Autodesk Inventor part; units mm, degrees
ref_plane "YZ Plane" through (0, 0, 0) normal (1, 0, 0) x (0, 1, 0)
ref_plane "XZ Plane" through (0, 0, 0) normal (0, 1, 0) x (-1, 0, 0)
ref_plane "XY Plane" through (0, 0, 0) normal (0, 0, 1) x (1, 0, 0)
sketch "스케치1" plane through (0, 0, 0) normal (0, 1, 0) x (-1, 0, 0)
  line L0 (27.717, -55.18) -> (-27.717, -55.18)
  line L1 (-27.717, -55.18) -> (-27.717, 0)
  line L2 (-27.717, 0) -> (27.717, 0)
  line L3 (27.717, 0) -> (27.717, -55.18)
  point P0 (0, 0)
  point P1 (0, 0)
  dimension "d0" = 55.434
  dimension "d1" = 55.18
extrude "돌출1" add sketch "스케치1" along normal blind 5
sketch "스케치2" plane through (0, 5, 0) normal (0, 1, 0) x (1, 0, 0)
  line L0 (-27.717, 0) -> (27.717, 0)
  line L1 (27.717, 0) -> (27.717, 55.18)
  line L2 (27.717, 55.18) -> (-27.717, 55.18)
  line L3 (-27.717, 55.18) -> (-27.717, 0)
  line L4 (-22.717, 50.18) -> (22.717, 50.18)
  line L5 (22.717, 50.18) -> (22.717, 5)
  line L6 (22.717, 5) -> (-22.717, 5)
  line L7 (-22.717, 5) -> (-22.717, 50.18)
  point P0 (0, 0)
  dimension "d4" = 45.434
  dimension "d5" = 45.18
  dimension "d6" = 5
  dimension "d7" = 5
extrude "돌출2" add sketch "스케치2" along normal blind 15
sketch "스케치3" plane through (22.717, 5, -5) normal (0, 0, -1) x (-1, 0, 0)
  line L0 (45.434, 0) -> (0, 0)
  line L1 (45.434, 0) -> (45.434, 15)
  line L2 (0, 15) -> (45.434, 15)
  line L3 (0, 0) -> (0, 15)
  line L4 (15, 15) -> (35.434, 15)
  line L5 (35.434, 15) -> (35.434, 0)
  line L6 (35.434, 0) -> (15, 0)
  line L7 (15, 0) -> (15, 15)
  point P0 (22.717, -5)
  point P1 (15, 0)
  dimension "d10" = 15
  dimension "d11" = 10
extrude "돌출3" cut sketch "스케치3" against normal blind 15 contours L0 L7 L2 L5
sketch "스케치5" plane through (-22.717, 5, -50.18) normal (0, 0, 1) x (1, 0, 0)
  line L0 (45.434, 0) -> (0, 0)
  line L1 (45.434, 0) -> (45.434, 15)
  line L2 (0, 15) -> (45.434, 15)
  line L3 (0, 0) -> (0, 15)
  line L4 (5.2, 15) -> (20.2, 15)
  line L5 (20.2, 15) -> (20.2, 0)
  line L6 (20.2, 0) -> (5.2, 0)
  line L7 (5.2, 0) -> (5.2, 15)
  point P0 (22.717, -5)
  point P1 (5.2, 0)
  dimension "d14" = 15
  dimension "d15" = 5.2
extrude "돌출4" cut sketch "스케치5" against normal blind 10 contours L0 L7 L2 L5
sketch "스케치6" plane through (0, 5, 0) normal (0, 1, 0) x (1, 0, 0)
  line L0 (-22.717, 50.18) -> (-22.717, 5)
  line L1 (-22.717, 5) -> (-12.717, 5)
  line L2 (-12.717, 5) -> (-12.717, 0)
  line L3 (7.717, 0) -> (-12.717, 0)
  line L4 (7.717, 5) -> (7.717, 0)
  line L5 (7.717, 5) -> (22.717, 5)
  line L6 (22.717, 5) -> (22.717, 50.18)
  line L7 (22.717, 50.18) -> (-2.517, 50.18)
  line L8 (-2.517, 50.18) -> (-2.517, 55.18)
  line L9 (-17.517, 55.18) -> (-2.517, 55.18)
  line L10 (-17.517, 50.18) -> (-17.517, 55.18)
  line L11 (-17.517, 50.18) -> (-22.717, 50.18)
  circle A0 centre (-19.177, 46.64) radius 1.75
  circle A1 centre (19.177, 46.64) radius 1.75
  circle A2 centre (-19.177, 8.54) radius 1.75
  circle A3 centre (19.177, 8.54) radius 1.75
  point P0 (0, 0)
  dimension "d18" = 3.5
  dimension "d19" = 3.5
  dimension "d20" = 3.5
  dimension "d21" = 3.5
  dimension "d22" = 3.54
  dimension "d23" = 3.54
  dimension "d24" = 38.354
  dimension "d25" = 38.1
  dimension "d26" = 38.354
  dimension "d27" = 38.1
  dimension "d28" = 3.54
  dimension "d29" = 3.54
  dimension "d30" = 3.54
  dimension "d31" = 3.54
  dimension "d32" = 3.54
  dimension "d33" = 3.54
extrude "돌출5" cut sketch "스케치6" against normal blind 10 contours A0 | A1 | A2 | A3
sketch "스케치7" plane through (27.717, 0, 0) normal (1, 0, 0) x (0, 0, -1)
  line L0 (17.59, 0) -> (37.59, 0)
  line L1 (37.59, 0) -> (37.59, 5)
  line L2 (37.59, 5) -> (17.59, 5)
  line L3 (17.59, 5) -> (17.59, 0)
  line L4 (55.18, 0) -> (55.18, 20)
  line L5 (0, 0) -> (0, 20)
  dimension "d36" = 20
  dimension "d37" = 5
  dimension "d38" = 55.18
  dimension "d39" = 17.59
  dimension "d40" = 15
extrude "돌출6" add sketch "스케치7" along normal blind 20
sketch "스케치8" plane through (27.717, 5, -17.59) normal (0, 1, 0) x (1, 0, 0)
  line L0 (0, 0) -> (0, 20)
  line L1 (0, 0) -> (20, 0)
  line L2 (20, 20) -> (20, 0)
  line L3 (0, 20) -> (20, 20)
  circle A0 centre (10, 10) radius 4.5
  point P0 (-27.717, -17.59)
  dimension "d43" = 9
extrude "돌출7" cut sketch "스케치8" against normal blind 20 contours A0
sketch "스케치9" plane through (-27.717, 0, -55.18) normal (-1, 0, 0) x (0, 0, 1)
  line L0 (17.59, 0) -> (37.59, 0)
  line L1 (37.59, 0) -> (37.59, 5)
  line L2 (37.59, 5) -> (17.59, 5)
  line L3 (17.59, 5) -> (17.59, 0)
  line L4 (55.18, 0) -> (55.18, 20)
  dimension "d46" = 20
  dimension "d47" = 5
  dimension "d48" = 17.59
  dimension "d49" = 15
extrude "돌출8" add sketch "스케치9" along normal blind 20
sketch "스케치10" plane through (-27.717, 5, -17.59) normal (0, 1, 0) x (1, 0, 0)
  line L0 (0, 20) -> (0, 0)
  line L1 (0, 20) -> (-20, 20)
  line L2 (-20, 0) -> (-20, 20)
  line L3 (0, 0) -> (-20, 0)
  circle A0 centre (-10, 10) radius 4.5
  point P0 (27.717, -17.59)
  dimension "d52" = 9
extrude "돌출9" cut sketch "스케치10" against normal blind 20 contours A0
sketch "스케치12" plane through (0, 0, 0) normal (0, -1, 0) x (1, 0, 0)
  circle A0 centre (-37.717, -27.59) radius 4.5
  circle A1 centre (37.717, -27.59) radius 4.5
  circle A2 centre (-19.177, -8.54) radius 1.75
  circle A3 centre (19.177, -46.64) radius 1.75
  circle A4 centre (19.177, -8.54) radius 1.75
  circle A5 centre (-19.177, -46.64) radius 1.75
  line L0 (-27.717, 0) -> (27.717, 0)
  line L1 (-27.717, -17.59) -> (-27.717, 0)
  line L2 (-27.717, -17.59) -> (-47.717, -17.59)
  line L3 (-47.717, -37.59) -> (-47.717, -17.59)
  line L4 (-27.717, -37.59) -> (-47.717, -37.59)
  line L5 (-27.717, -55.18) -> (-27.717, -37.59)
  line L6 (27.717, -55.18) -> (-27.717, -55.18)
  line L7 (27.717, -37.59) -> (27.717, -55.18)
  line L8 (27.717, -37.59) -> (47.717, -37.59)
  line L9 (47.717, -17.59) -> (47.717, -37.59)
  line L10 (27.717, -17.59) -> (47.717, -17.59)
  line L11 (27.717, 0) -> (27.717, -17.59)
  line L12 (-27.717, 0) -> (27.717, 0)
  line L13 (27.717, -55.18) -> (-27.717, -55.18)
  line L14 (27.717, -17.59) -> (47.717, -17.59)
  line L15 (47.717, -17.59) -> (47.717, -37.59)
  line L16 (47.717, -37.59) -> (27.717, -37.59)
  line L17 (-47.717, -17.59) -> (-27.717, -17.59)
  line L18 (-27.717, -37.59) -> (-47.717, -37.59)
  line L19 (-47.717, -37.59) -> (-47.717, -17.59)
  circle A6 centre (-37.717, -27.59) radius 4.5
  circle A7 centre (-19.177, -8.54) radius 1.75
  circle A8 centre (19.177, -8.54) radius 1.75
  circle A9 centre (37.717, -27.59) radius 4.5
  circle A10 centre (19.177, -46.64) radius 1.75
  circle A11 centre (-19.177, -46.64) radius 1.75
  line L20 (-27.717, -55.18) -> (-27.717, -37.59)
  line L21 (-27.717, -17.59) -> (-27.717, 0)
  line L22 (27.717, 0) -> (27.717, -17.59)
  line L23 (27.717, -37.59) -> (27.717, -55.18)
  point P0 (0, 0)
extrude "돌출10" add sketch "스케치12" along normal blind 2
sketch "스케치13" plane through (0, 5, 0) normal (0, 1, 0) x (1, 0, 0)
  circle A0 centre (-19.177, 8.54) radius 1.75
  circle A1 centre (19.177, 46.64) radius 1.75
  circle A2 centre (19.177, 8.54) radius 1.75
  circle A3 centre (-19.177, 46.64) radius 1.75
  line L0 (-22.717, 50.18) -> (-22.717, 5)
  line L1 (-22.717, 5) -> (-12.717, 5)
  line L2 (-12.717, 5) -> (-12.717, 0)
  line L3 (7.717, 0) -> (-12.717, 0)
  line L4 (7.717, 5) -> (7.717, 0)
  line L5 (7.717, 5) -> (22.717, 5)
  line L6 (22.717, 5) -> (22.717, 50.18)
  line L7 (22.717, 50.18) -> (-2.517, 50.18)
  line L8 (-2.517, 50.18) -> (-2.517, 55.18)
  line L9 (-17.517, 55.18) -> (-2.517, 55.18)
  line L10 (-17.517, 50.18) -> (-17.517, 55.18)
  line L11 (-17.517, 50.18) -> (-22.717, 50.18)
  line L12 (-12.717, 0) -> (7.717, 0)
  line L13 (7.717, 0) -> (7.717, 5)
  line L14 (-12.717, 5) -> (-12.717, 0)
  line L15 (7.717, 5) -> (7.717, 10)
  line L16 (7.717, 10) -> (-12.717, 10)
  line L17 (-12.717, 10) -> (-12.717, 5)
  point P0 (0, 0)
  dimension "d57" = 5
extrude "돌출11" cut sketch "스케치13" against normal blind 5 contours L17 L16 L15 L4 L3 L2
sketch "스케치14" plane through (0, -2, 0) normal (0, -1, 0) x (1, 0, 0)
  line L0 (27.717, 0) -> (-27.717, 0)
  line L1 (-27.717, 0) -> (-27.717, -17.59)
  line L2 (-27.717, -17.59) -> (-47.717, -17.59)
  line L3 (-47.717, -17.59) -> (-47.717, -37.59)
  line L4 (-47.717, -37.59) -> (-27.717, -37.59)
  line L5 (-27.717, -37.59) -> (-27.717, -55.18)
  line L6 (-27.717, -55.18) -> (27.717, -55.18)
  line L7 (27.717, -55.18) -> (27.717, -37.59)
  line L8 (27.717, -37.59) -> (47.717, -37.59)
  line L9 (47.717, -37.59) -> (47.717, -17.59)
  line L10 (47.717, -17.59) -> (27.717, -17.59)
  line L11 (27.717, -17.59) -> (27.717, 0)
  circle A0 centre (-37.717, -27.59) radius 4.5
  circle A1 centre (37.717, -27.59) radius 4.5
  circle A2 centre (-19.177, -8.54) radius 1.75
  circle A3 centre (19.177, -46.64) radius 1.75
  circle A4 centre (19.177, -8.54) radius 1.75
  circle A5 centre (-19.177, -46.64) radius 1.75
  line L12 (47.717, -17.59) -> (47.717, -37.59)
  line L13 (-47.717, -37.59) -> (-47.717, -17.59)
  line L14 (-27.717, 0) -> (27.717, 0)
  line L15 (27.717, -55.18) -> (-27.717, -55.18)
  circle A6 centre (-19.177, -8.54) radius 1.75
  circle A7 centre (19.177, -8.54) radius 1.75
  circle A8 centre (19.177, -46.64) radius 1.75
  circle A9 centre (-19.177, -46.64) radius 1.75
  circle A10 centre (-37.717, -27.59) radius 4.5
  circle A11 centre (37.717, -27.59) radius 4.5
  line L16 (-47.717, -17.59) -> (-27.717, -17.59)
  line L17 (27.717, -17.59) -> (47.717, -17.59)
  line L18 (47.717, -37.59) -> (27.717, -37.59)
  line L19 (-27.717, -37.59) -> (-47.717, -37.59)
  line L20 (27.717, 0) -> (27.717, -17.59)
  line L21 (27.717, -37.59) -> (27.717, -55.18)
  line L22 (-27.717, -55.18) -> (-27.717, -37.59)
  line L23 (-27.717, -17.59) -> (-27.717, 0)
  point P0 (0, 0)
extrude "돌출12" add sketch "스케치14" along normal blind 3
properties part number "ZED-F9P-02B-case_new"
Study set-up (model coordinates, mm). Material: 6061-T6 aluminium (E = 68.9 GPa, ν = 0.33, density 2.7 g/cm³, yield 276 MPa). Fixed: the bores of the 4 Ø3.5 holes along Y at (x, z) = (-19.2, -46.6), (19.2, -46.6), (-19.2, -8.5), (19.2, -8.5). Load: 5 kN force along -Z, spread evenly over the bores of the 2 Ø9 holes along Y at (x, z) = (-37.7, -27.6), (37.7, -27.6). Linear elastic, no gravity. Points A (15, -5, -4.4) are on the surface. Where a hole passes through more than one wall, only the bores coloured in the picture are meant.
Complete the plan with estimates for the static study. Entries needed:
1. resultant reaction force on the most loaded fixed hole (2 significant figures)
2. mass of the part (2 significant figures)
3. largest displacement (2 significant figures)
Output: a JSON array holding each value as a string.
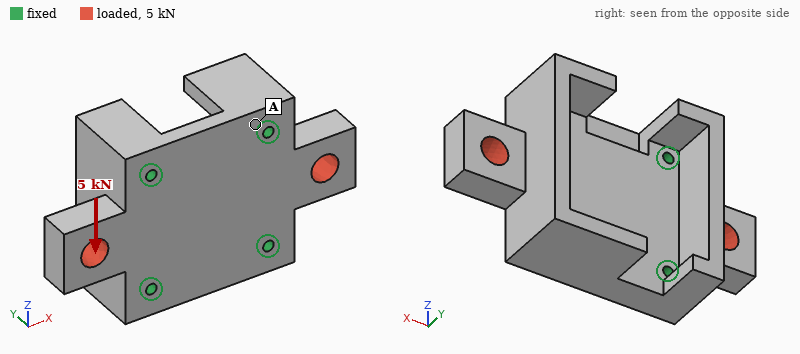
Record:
["1.6 kN", "130 g", "30 µm"]
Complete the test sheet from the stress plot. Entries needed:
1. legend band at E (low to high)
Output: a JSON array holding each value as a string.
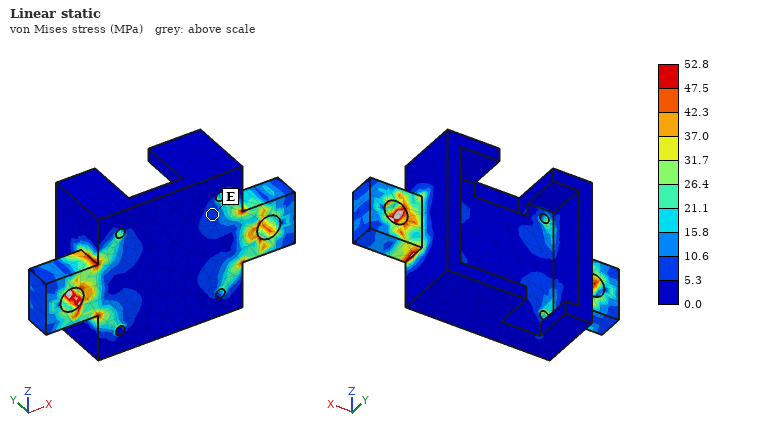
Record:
["5.3 to 10.6 MPa"]
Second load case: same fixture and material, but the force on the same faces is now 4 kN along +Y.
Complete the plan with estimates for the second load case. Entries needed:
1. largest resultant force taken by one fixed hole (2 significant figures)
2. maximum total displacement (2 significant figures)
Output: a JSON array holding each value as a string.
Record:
["1.1 kN", "87 µm"]
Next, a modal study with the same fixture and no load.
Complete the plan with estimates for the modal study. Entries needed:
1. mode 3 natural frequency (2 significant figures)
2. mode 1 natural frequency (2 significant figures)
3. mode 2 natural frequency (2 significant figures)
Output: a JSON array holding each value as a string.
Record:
["15 kHz", "8600 Hz", "9000 Hz"]
